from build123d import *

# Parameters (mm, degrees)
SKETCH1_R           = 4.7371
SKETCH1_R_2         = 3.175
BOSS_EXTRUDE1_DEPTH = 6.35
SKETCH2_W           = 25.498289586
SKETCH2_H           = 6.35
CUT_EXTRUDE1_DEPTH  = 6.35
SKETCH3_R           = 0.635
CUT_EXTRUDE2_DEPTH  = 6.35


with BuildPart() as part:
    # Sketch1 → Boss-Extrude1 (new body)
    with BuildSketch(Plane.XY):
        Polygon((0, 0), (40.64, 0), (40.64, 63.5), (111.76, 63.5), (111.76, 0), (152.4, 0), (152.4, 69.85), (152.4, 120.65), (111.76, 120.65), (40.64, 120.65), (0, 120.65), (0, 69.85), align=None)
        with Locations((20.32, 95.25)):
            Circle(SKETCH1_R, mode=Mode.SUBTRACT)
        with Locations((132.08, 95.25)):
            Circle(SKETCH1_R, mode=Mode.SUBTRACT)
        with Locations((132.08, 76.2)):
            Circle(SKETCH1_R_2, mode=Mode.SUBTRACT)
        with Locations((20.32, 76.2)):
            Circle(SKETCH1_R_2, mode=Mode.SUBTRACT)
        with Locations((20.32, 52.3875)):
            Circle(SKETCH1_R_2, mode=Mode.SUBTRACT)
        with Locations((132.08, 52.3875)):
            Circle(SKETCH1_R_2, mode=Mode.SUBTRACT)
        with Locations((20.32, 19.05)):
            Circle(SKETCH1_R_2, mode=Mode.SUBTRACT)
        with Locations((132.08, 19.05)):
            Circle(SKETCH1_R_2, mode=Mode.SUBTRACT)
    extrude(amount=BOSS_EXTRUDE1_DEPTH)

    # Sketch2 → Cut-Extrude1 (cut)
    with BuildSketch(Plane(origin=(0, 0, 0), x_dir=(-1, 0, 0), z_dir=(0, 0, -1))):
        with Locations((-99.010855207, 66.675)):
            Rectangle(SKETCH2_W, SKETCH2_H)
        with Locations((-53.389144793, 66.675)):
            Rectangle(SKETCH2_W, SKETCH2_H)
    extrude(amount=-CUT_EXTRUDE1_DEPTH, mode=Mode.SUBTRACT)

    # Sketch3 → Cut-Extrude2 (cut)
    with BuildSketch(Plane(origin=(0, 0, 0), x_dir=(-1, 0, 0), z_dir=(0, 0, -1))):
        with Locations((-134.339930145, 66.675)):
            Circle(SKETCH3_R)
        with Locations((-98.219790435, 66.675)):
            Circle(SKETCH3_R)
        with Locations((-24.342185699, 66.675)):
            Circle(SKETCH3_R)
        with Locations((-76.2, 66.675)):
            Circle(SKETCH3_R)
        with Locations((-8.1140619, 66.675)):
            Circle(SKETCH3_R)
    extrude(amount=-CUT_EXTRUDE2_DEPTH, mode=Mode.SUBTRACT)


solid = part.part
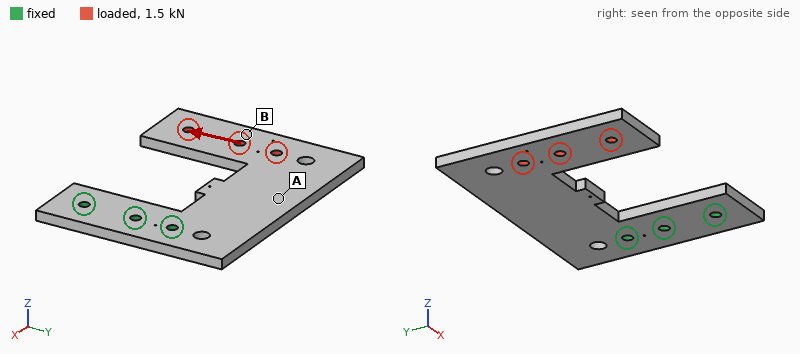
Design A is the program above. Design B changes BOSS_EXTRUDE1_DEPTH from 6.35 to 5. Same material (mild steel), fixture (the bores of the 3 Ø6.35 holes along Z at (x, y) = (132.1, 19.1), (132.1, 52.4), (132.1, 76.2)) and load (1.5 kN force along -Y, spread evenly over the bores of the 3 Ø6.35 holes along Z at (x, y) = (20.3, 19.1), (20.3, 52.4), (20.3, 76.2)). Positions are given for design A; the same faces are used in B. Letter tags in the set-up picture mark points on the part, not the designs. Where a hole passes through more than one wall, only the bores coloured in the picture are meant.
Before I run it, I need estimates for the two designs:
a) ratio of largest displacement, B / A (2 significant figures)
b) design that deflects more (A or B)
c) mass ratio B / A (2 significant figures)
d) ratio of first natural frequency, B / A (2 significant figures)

1.3
B
0.79
0.80
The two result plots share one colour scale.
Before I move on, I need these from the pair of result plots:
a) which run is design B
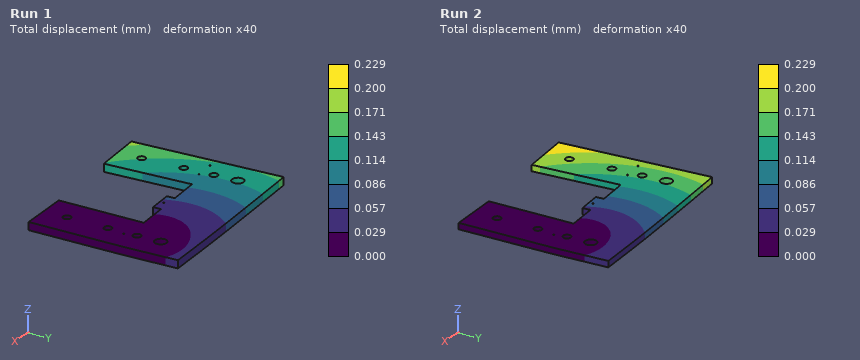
Run 2
